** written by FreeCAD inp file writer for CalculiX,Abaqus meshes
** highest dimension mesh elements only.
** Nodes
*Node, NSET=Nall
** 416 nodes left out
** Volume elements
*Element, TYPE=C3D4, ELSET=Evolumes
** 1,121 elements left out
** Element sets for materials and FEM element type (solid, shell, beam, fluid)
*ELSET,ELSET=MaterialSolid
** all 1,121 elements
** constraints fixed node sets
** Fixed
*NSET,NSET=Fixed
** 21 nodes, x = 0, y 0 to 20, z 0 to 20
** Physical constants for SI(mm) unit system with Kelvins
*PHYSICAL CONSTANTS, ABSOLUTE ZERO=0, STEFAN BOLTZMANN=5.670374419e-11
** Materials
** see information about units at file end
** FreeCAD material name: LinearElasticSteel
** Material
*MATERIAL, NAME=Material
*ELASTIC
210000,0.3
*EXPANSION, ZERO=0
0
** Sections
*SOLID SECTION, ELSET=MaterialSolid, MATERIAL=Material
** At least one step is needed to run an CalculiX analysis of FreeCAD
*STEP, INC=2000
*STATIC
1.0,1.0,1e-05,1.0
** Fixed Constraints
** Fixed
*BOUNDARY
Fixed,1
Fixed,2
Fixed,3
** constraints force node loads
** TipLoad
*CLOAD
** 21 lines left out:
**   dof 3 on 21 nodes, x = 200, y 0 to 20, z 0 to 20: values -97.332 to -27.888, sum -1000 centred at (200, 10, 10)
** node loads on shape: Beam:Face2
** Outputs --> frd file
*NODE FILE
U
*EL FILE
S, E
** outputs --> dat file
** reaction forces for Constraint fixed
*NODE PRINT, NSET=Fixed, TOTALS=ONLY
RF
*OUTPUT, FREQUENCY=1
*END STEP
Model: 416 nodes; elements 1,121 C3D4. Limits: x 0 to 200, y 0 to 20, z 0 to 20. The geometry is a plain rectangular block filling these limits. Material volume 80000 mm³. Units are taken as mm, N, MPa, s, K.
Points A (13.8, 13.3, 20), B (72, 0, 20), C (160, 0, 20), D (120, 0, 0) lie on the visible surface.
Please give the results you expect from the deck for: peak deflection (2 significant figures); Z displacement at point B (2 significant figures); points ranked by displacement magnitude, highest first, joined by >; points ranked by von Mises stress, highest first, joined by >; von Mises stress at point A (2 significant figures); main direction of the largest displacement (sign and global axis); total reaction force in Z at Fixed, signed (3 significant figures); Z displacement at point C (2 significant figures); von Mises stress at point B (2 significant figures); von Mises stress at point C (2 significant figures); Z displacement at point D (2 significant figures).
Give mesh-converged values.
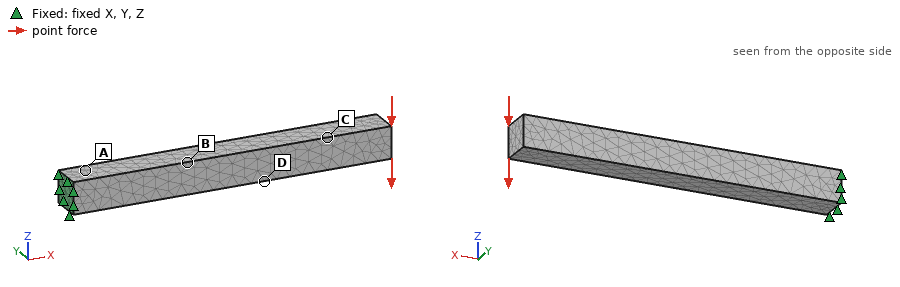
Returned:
0.96 mm
-0.16 mm
C > D > B > A
A > B > D > C
140 MPa
-Z
1000 N
-0.67 mm
96 MPa
30 MPa
-0.41 mm
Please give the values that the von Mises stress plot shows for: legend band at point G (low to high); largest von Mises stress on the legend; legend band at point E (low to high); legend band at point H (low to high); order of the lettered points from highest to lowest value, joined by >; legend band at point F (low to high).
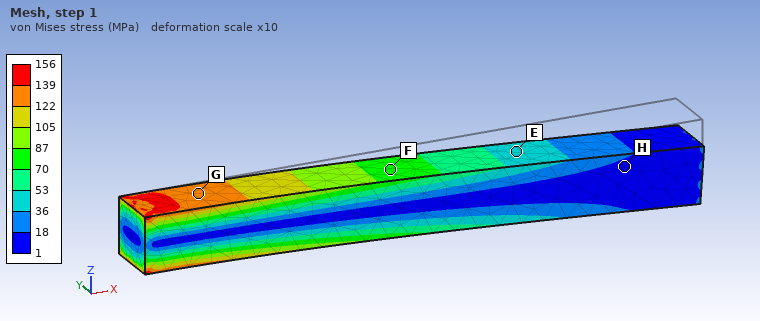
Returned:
122 to 139 MPa
156 MPa
36 to 53 MPa
1 to 18 MPa
G > F > E > H
70 to 87 MPa
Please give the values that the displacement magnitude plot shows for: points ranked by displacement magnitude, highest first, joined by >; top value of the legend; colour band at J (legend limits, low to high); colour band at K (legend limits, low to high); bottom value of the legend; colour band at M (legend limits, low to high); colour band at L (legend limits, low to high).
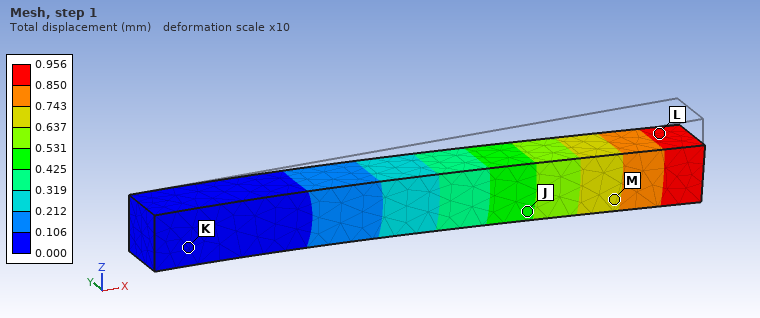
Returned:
L > M > J > K
0.956 mm
0.425 to 0.531 mm
0.000 to 0.106 mm
0.000 mm
0.637 to 0.743 mm
0.850 to 0.956 mm
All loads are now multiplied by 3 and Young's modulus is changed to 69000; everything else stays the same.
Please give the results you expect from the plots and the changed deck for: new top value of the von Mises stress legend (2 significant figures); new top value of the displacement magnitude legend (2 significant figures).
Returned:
470 MPa
8.7 mm
